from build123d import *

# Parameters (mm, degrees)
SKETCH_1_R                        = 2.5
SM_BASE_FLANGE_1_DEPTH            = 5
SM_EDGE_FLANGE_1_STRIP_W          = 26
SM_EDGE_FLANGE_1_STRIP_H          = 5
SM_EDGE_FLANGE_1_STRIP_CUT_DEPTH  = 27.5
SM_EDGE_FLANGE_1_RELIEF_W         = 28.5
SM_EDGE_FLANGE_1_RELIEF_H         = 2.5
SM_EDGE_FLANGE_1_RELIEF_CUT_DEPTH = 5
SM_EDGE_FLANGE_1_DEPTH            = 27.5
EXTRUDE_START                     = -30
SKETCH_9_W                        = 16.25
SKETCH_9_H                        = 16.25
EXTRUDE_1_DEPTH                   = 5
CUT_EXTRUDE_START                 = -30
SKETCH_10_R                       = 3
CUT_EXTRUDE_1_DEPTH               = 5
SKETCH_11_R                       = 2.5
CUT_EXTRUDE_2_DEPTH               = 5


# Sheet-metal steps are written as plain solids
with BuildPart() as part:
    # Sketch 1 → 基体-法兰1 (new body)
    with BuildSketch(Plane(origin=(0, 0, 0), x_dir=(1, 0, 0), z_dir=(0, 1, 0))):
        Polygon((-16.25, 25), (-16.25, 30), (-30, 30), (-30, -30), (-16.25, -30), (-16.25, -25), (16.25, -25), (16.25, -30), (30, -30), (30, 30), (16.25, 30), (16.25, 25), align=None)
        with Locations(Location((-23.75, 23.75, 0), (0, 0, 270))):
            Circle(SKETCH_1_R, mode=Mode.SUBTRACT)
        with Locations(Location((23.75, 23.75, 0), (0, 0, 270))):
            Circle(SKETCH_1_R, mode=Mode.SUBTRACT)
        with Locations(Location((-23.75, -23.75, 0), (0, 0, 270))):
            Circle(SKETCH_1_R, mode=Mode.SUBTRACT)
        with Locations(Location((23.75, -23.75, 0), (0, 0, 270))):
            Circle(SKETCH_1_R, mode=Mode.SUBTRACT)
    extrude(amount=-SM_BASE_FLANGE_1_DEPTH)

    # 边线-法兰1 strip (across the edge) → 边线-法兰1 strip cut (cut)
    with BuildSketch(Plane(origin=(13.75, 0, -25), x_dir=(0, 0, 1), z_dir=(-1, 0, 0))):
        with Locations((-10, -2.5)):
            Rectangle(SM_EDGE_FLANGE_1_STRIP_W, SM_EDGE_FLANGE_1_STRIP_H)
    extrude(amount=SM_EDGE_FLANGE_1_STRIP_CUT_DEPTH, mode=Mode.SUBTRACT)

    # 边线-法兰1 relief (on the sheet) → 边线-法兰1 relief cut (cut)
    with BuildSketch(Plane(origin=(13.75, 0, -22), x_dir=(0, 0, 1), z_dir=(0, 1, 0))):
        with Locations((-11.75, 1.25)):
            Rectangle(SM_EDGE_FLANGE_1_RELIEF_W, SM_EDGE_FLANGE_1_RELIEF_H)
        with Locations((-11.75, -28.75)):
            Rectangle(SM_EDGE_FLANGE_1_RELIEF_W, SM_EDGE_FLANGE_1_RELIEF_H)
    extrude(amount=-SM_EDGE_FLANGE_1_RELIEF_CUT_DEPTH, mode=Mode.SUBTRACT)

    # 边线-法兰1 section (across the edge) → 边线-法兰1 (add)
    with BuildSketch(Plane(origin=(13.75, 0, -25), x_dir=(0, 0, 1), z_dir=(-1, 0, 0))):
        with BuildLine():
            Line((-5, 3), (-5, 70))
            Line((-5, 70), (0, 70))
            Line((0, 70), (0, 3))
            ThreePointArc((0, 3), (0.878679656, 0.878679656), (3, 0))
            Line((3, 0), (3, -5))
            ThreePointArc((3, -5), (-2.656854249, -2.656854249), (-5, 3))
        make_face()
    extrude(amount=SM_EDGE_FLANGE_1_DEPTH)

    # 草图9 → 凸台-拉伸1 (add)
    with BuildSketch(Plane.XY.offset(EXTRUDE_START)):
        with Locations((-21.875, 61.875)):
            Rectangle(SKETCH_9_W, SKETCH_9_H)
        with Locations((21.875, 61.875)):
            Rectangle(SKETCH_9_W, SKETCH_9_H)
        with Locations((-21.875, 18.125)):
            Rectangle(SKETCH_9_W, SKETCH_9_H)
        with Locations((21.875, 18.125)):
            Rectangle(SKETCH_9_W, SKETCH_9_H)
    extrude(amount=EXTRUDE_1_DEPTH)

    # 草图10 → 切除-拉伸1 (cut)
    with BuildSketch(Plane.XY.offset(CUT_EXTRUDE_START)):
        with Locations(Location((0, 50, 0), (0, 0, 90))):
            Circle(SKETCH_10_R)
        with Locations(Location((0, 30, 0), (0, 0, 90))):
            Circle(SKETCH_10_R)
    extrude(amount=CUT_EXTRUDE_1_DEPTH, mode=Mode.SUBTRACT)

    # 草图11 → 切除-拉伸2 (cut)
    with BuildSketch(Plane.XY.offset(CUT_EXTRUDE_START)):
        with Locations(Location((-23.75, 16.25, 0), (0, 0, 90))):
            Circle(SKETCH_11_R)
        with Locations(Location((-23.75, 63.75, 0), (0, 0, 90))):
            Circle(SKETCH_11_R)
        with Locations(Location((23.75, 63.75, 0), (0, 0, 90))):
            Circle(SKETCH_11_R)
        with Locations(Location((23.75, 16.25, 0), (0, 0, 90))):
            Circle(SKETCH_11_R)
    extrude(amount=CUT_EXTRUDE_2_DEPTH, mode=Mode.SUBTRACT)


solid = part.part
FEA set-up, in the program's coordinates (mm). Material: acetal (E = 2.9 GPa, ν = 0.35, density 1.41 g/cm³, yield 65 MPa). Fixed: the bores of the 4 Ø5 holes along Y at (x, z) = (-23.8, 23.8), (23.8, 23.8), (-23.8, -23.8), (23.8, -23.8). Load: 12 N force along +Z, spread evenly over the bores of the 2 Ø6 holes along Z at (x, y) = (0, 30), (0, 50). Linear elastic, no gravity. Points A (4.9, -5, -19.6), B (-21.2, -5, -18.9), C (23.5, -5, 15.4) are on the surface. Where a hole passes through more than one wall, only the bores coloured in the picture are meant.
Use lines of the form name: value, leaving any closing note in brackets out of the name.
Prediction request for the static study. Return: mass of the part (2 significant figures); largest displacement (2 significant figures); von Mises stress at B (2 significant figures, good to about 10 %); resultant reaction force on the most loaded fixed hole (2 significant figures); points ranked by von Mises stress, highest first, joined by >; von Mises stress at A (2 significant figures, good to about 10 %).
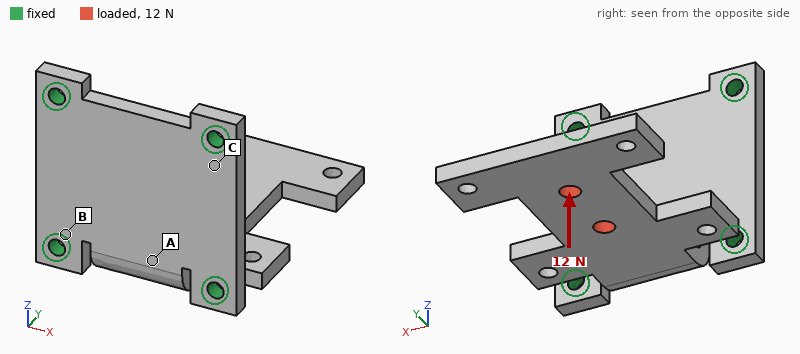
mass of the part: 43 g
largest displacement: 1.3 mm
von Mises stress at B: 1.1 MPa
resultant reaction force on the most loaded fixed hole: 7.2 N
points ranked by von Mises stress, highest first, joined by >: A > B > C
von Mises stress at A: 3.2 MPa
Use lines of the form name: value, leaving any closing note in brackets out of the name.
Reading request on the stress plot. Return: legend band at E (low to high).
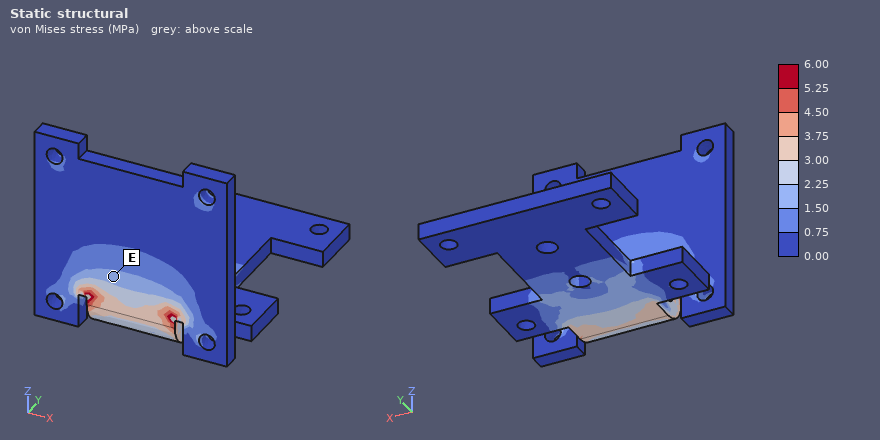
legend band at E: 1.50 to 2.25 MPa
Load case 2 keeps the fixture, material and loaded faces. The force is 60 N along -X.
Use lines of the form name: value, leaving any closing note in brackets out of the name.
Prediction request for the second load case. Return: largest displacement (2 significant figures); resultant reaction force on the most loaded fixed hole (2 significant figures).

largest displacement: 1.4 mm
resultant reaction force on the most loaded fixed hole: 75 N
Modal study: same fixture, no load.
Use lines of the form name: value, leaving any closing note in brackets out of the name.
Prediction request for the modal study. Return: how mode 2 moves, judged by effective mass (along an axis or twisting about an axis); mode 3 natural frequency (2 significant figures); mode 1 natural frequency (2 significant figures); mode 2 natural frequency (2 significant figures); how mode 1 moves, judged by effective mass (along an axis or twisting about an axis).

how mode 2 moves, judged by effective mass: along X
mode 3 natural frequency: 470 Hz
mode 1 natural frequency: 130 Hz
mode 2 natural frequency: 290 Hz
how mode 1 moves, judged by effective mass: along Z
